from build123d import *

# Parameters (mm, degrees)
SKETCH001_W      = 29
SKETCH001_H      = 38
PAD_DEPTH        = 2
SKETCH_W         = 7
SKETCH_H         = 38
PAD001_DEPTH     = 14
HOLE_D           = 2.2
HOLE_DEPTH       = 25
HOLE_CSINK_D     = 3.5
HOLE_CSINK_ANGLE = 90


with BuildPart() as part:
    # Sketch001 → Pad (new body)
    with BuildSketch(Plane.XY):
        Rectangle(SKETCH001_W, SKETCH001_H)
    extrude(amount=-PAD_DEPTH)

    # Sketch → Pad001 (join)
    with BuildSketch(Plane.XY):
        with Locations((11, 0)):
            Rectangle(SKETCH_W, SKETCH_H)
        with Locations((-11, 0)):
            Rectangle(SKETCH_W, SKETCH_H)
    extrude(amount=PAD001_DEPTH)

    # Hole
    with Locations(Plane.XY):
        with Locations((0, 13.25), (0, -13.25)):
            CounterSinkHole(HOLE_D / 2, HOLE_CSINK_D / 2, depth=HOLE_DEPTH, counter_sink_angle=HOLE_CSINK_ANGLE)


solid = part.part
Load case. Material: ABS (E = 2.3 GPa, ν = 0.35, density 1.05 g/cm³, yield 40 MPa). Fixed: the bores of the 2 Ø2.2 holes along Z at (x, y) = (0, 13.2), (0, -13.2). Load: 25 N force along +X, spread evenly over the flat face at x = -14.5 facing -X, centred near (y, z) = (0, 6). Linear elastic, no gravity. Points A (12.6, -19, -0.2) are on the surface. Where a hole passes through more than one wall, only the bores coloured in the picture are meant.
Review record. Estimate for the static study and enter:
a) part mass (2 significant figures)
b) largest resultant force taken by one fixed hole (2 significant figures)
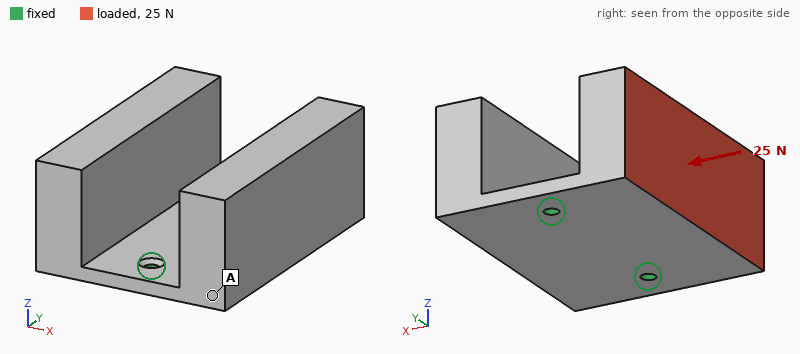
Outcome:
10 g
13 N
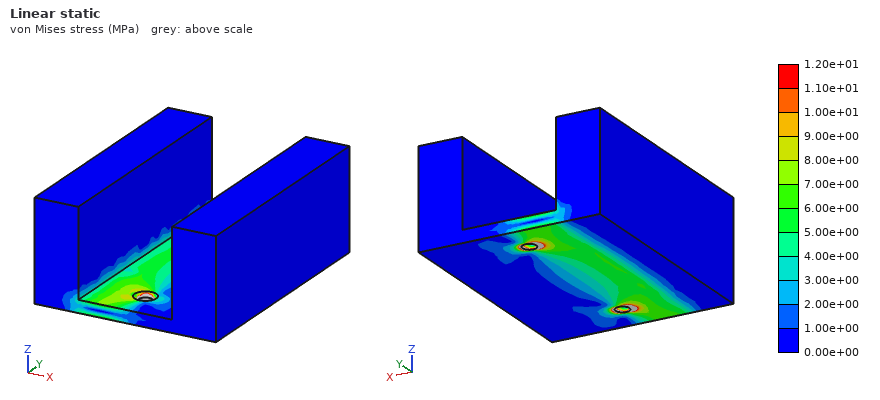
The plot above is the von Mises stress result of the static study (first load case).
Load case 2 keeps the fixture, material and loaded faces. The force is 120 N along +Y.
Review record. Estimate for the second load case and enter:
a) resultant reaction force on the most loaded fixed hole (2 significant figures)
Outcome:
93 N
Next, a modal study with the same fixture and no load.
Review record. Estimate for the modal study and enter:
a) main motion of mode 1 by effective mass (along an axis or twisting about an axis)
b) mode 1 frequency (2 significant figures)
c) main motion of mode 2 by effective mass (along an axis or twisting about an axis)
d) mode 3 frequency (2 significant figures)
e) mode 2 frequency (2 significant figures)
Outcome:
along X
410 Hz
along Z
1500 Hz
590 Hz
